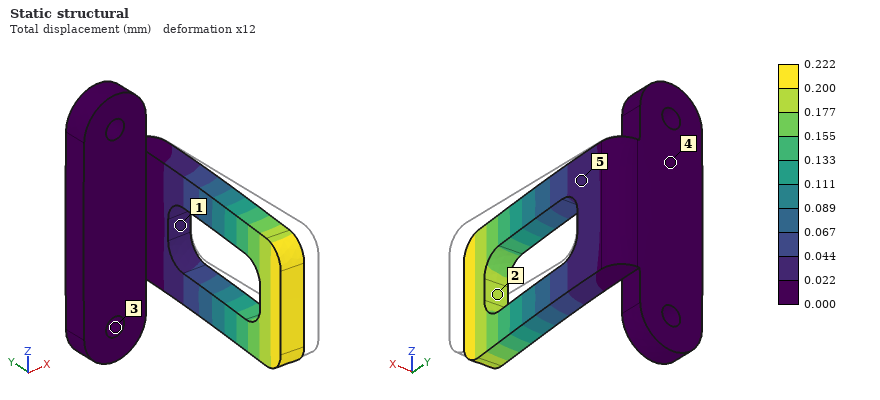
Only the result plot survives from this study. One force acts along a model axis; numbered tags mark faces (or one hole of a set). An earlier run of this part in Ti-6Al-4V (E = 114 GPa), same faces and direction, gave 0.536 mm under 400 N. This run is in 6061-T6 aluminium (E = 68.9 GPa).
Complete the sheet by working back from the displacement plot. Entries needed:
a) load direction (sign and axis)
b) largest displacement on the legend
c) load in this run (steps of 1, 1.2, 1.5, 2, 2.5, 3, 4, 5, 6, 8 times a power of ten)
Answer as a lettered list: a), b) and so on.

a) -X
b) 0.222 mm
c) 100 N
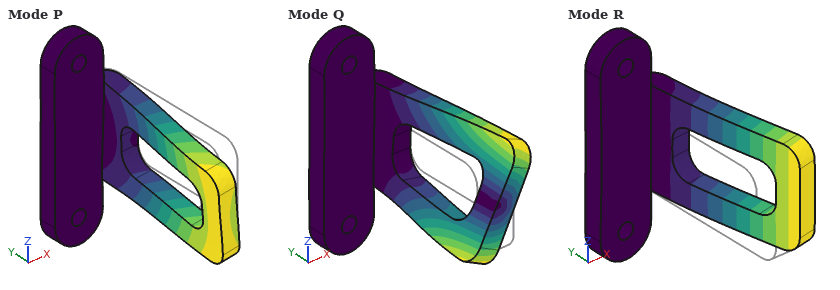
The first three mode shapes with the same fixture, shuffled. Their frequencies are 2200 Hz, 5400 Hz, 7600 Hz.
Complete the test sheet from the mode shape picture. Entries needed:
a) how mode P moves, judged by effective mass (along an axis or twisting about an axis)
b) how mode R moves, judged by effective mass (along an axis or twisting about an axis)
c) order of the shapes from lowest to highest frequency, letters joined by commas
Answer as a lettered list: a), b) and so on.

a) along Z
b) along X
c) R, P, Q
